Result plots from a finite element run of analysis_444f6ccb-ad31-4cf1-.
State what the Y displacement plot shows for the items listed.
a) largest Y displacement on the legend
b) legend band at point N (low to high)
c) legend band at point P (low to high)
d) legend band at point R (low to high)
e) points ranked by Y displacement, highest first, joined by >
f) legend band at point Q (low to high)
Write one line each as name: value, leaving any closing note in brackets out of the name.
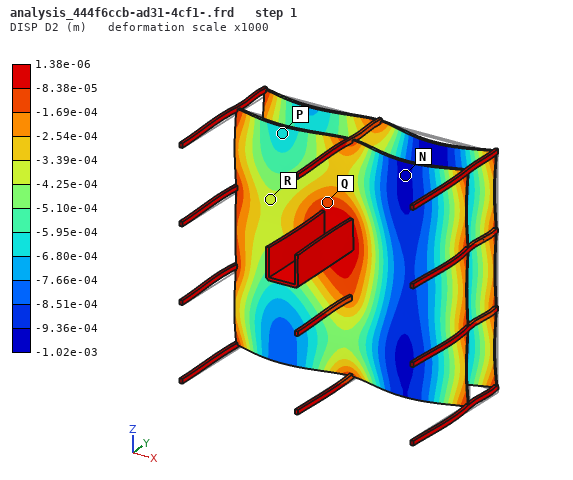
largest Y displacement on the legend: 1.38e-06 m
legend band at point N: -1.02e-03 to -9.36e-04 m
legend band at point P: -6.80e-04 to -5.95e-04 m
legend band at point R: -4.25e-04 to -3.39e-04 m
points ranked by Y displacement, highest first, joined by >: Q > R > P > N
legend band at point Q: -1.69e-04 to -8.38e-05 m
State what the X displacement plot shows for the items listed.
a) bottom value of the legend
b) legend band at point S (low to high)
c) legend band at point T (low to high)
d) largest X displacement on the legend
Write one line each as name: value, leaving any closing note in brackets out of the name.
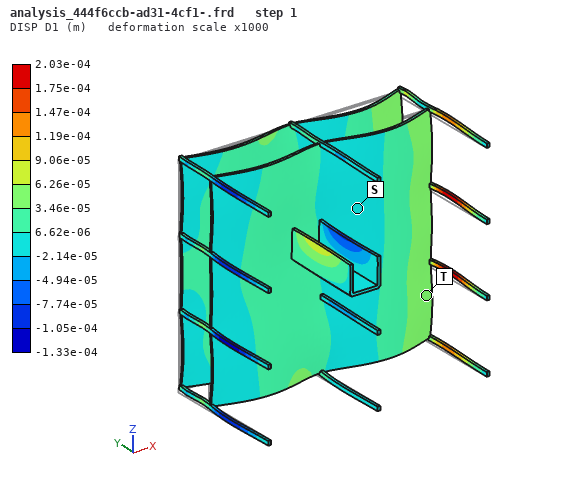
bottom value of the legend: -1.33e-04 m
legend band at point S: -2.14e-05 to 6.62e-06 m
legend band at point T: 3.46e-05 to 6.26e-05 m
largest X displacement on the legend: 2.03e-04 m
